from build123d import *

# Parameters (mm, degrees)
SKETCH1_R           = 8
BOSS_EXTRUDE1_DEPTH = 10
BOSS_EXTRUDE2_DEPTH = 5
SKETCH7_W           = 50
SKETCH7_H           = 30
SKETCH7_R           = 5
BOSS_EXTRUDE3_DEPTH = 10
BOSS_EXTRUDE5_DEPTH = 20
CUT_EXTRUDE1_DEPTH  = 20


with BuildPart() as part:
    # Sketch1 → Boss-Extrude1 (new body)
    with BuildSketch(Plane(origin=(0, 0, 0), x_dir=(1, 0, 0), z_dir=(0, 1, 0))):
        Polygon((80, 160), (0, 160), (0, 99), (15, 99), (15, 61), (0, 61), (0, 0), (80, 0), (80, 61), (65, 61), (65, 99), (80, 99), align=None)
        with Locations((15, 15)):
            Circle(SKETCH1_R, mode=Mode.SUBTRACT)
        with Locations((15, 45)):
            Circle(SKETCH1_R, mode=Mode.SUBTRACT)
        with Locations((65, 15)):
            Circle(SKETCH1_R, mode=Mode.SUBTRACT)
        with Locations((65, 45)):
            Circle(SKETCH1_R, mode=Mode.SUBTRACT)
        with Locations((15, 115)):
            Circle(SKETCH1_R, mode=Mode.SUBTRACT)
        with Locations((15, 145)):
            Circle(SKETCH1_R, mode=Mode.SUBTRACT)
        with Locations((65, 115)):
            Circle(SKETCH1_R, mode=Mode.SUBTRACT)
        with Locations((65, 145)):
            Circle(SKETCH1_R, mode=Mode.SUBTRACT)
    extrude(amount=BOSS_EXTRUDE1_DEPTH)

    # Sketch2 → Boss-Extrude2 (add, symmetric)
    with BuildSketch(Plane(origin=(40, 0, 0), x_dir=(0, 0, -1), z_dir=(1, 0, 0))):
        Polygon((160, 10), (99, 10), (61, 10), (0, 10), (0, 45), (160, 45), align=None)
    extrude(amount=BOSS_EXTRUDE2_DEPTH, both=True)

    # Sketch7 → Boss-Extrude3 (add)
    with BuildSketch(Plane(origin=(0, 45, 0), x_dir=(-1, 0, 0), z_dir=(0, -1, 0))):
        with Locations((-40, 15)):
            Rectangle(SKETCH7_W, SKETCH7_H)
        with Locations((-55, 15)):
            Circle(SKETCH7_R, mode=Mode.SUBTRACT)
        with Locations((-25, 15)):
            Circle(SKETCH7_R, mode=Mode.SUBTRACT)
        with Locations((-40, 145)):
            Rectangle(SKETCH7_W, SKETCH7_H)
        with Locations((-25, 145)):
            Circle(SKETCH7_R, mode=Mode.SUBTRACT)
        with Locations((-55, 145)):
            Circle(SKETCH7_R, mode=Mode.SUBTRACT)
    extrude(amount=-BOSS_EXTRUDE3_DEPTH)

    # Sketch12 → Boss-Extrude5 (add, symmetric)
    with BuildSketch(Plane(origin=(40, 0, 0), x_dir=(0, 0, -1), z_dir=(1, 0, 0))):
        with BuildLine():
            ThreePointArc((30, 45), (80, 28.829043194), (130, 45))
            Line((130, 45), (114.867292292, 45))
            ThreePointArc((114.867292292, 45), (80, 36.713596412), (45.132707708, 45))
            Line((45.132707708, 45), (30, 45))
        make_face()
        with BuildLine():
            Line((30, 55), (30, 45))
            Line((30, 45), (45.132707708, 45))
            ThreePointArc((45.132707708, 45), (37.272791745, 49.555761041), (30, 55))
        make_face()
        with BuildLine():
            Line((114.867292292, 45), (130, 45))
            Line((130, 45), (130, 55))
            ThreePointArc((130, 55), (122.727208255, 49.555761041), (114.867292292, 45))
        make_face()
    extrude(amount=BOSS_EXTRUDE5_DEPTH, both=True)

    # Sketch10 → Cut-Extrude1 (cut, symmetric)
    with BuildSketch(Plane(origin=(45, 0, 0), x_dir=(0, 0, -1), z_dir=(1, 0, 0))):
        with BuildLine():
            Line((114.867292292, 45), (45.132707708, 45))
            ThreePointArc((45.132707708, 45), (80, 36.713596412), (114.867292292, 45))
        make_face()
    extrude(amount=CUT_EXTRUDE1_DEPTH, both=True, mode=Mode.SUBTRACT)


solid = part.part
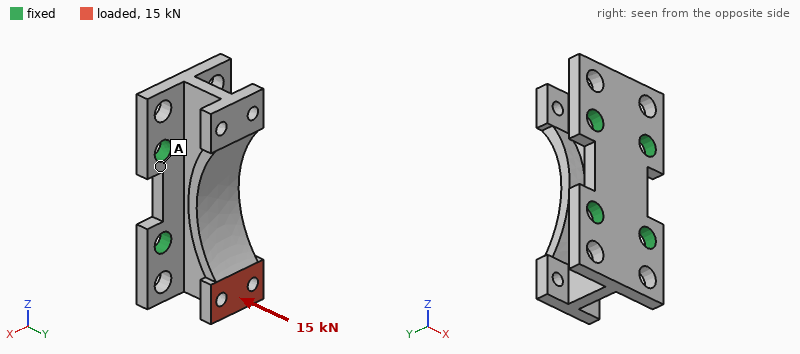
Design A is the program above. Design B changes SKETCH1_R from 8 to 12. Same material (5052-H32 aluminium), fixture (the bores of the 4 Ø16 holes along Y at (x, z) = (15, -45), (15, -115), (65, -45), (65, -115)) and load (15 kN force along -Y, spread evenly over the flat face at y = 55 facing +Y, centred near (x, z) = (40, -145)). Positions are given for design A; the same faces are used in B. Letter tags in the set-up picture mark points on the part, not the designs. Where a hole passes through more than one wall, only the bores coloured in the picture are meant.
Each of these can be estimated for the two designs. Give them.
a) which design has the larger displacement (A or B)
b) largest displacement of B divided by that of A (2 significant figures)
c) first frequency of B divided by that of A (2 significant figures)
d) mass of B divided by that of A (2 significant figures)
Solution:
A
0.87
1.0
0.90
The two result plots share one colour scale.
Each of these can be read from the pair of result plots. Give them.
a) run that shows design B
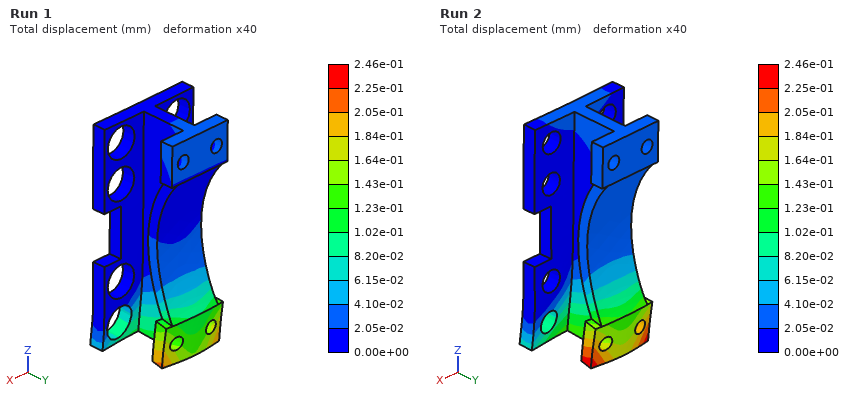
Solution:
Run 1
